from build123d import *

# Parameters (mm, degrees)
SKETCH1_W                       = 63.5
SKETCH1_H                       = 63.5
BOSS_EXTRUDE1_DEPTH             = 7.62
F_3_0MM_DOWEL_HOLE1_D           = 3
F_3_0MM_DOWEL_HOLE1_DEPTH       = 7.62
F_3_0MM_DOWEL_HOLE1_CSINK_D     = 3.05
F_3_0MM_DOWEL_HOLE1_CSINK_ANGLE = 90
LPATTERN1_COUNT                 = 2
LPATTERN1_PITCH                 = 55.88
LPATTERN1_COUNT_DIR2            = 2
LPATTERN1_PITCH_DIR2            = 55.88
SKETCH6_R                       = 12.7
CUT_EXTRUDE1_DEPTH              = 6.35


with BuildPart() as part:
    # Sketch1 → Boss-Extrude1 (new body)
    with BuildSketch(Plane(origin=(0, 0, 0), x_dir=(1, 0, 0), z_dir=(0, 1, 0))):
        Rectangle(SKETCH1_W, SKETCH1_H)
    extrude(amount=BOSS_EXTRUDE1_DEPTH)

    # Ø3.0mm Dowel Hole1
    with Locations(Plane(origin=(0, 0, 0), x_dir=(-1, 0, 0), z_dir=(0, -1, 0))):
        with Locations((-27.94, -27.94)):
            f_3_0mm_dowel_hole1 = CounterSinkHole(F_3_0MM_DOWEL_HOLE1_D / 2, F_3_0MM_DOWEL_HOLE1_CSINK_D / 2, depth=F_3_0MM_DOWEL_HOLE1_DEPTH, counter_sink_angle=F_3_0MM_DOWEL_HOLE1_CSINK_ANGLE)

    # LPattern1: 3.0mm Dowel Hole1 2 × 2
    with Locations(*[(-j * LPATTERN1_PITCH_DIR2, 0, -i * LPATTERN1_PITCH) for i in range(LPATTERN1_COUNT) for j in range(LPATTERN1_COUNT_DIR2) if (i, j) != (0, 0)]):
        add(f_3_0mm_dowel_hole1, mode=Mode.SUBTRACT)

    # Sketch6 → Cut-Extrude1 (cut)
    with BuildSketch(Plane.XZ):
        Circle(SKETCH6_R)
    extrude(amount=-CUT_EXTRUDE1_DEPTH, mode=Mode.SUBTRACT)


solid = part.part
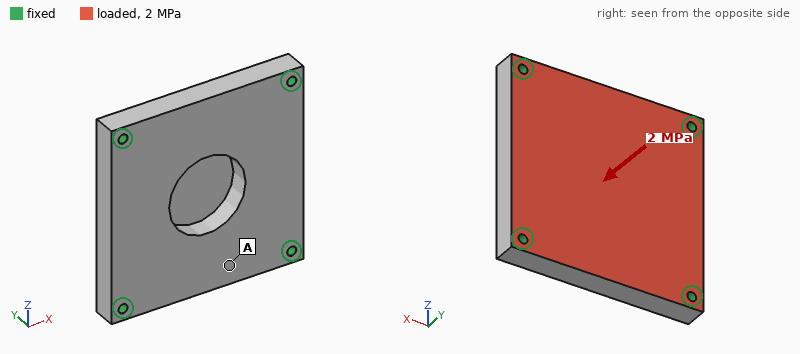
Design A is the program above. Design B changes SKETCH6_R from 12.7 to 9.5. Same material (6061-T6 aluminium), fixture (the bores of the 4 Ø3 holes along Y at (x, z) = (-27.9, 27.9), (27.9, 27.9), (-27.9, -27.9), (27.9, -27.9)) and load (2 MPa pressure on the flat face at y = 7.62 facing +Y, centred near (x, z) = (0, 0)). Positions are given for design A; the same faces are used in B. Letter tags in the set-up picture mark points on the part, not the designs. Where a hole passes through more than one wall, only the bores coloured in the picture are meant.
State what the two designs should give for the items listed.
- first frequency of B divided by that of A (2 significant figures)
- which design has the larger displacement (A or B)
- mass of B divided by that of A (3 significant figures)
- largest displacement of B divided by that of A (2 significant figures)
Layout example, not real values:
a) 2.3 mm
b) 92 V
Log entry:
a) 0.97
b) A
c) 1.05
d) 0.70
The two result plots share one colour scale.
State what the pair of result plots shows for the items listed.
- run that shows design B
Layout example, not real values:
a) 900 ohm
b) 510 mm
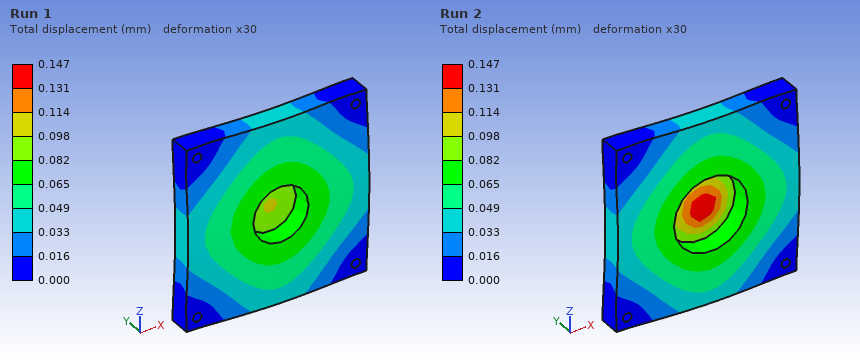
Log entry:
a) Run 1
